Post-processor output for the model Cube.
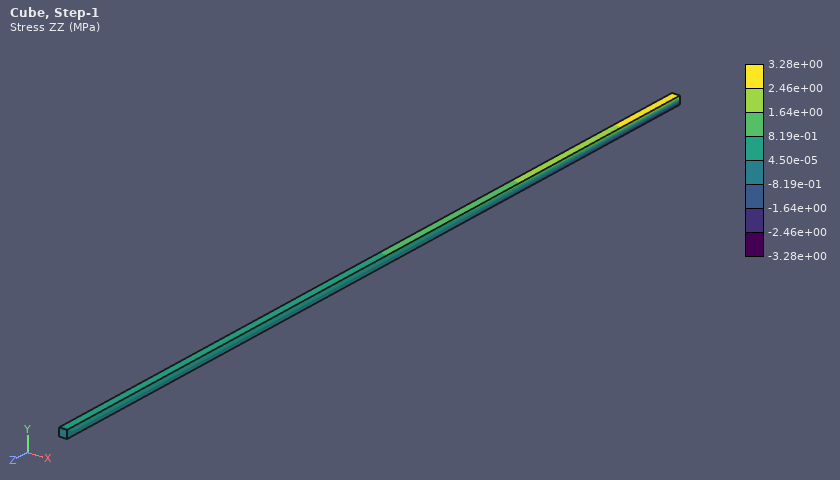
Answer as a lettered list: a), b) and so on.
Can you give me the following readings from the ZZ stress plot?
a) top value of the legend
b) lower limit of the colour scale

a) 3.28e+00 MPa
b) -3.28e+00 MPa
